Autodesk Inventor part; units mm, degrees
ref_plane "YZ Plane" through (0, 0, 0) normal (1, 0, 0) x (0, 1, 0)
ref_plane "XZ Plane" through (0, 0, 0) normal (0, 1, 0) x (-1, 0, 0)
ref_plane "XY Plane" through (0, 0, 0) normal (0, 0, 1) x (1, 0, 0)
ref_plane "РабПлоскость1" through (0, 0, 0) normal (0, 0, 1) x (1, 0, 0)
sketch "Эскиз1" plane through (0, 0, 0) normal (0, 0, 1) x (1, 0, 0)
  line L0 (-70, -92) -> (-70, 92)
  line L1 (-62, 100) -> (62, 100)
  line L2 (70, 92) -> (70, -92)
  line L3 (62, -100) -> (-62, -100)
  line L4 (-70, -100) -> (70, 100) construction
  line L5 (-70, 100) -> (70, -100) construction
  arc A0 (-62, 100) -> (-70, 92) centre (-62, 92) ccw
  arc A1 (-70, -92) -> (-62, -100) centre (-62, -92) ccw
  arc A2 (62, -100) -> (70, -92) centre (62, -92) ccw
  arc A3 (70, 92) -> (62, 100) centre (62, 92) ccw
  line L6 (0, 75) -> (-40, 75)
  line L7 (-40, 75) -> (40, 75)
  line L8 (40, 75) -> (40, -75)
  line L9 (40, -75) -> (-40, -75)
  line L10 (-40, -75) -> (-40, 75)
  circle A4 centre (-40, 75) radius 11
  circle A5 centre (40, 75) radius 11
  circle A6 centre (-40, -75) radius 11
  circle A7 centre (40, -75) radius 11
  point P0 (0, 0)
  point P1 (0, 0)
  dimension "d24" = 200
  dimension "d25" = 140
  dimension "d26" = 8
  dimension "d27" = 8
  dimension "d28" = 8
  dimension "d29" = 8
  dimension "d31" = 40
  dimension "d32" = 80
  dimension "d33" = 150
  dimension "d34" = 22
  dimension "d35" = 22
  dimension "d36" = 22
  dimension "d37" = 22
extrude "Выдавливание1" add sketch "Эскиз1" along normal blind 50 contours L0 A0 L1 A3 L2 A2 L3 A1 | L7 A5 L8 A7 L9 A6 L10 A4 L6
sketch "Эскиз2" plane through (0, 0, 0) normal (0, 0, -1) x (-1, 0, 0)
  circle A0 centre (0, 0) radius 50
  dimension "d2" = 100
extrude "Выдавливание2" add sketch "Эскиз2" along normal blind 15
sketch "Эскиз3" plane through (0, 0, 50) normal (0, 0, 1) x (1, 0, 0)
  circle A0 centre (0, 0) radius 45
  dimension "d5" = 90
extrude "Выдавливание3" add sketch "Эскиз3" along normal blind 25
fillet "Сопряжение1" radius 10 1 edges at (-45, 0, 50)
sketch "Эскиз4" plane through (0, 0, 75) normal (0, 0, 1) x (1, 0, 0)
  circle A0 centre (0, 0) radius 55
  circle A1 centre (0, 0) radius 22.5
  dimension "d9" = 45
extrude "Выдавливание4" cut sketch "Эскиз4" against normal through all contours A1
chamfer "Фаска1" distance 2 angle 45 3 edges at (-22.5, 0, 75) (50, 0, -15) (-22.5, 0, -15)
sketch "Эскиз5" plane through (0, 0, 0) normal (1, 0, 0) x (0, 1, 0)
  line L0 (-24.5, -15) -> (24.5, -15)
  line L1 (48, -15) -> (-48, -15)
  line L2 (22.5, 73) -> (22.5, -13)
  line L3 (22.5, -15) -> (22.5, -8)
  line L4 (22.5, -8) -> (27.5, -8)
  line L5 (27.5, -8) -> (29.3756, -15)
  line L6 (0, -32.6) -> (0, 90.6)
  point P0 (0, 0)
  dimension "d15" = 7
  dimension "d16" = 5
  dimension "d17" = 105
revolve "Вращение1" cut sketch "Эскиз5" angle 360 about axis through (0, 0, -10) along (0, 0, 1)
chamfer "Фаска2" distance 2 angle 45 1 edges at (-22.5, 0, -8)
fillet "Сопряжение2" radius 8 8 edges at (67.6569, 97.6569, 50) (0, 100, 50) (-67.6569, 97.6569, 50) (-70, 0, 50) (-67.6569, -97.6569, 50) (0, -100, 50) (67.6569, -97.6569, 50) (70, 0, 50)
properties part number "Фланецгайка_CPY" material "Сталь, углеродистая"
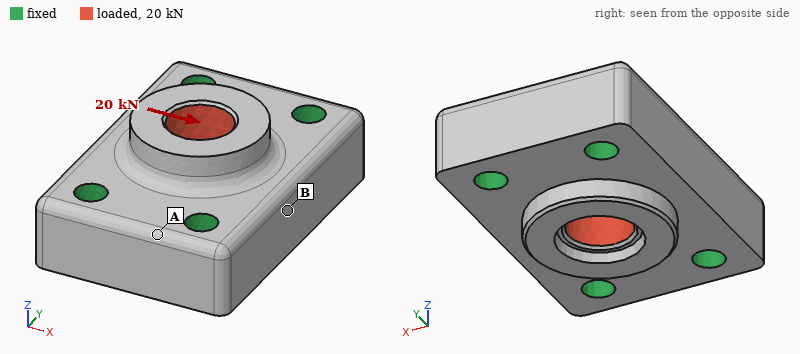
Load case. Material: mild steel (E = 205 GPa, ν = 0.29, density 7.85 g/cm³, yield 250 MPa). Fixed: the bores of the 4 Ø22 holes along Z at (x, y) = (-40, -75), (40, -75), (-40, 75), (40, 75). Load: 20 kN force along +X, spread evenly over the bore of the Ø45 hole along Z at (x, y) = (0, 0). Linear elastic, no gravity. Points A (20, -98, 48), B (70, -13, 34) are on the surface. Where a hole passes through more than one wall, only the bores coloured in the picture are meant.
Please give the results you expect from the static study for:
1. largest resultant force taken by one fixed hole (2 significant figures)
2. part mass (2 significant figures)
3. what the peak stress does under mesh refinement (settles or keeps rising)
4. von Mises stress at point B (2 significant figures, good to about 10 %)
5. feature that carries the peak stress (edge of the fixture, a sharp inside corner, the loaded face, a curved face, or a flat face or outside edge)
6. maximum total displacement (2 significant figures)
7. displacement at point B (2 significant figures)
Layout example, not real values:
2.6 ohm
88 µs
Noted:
5.8 kN
11 kg
keeps rising
2.4 MPa
edge of the fixture
1.9 µm
1.2 µm
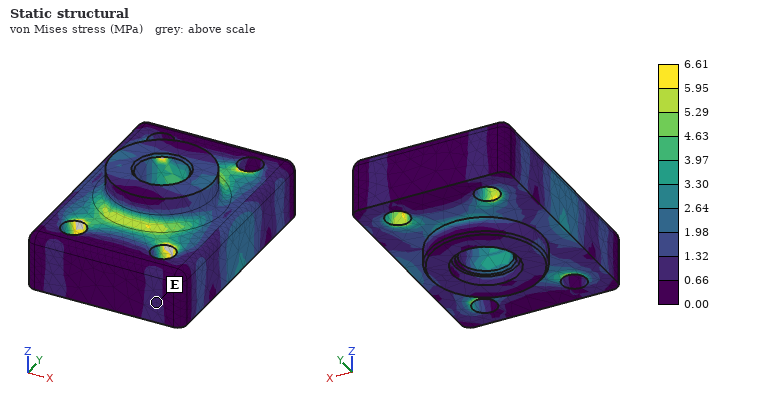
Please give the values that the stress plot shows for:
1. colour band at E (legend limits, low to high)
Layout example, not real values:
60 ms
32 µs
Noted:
0.66 to 1.32 MPa
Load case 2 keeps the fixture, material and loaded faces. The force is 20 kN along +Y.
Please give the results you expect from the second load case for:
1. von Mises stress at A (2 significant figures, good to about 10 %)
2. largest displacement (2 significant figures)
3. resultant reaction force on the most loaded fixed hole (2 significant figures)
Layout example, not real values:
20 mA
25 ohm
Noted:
0.49 MPa
1.1 µm
5.2 kN
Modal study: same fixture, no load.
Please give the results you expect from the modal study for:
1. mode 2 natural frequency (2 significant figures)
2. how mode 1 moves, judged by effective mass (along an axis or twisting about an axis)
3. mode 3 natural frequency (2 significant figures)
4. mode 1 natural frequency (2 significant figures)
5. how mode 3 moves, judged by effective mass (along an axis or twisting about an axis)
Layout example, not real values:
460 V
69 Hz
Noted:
8100 Hz
along Z
9200 Hz
7600 Hz
along X
